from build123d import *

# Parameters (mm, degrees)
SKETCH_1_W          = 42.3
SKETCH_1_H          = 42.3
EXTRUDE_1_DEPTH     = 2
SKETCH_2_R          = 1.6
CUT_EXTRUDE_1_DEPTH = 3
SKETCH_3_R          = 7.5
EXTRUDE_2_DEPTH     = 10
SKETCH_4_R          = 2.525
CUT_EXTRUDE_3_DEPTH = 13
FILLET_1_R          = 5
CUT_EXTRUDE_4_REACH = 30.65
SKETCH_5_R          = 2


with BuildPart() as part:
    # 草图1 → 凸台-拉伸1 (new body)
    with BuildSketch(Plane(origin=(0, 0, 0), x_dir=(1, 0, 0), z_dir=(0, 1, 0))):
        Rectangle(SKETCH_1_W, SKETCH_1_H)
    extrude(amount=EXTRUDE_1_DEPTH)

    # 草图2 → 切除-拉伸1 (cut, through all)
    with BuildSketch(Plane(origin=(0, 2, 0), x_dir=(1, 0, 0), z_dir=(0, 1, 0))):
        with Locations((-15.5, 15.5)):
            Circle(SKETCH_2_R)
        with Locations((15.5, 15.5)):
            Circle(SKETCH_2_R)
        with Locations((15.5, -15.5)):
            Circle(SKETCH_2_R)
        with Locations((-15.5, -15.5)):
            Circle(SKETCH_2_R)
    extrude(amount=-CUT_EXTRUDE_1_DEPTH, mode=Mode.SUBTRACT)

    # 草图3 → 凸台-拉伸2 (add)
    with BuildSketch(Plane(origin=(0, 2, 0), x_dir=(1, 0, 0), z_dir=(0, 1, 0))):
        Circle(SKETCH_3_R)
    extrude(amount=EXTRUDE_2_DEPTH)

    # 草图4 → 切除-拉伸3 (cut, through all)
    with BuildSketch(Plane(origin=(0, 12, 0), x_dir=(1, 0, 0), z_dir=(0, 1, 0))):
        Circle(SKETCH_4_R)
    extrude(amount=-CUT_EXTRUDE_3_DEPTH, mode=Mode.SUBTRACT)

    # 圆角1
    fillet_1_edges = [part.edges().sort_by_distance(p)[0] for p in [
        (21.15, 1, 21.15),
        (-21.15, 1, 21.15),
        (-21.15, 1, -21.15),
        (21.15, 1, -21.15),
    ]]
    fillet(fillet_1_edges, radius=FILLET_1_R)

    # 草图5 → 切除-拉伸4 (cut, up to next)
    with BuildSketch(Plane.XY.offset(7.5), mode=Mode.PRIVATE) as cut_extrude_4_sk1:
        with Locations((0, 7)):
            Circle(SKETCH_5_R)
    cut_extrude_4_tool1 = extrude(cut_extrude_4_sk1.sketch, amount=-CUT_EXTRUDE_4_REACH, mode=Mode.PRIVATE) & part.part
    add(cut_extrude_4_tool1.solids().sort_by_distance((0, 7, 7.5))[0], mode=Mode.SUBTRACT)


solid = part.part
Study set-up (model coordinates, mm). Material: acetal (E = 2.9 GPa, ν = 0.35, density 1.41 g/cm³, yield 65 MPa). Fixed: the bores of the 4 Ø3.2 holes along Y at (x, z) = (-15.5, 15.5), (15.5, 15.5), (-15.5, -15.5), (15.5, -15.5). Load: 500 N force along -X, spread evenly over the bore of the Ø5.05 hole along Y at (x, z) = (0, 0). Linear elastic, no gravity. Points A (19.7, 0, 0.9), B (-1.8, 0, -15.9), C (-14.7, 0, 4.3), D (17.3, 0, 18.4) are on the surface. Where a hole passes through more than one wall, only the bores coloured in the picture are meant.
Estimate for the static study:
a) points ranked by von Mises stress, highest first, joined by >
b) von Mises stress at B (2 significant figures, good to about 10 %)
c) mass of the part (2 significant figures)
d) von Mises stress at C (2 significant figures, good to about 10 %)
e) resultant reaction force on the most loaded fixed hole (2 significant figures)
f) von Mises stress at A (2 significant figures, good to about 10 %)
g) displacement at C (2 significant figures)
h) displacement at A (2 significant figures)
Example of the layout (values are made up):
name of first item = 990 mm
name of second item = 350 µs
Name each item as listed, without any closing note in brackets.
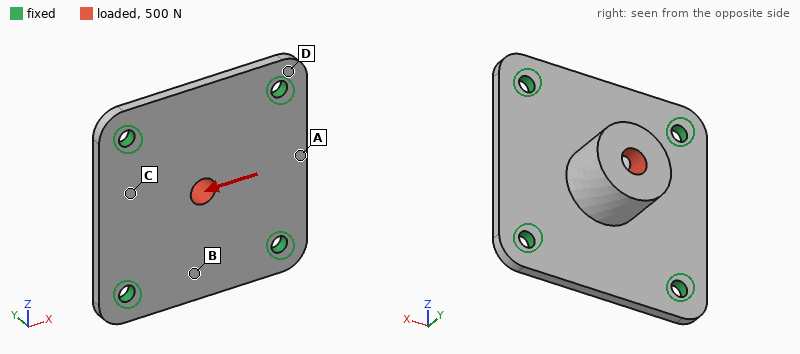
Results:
points ranked by von Mises stress, highest first, joined by > = A > C > B > D
von Mises stress at B = 7.4 MPa
mass of the part = 7.0 g
von Mises stress at C = 12 MPa
resultant reaction force on the most loaded fixed hole = 150 N
von Mises stress at A = 16 MPa
displacement at C = 0.26 mm
displacement at A = 0.23 mm
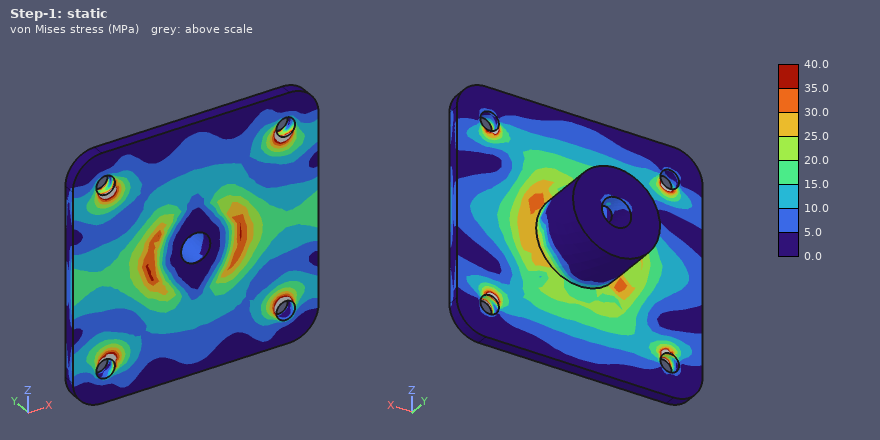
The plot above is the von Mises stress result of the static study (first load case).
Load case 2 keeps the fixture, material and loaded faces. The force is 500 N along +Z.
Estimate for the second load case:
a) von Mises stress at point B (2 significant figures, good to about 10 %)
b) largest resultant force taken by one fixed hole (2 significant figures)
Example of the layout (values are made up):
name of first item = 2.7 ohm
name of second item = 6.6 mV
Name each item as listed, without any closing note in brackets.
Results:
von Mises stress at point B = 15 MPa
largest resultant force taken by one fixed hole = 150 N
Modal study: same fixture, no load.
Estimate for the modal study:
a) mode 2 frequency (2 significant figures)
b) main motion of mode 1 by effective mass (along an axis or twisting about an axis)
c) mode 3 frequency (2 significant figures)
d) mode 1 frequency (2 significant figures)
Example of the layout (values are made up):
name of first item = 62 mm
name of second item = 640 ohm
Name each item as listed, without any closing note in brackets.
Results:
mode 2 frequency = 2600 Hz
main motion of mode 1 by effective mass = along Y
mode 3 frequency = 2600 Hz
mode 1 frequency = 1700 Hz
